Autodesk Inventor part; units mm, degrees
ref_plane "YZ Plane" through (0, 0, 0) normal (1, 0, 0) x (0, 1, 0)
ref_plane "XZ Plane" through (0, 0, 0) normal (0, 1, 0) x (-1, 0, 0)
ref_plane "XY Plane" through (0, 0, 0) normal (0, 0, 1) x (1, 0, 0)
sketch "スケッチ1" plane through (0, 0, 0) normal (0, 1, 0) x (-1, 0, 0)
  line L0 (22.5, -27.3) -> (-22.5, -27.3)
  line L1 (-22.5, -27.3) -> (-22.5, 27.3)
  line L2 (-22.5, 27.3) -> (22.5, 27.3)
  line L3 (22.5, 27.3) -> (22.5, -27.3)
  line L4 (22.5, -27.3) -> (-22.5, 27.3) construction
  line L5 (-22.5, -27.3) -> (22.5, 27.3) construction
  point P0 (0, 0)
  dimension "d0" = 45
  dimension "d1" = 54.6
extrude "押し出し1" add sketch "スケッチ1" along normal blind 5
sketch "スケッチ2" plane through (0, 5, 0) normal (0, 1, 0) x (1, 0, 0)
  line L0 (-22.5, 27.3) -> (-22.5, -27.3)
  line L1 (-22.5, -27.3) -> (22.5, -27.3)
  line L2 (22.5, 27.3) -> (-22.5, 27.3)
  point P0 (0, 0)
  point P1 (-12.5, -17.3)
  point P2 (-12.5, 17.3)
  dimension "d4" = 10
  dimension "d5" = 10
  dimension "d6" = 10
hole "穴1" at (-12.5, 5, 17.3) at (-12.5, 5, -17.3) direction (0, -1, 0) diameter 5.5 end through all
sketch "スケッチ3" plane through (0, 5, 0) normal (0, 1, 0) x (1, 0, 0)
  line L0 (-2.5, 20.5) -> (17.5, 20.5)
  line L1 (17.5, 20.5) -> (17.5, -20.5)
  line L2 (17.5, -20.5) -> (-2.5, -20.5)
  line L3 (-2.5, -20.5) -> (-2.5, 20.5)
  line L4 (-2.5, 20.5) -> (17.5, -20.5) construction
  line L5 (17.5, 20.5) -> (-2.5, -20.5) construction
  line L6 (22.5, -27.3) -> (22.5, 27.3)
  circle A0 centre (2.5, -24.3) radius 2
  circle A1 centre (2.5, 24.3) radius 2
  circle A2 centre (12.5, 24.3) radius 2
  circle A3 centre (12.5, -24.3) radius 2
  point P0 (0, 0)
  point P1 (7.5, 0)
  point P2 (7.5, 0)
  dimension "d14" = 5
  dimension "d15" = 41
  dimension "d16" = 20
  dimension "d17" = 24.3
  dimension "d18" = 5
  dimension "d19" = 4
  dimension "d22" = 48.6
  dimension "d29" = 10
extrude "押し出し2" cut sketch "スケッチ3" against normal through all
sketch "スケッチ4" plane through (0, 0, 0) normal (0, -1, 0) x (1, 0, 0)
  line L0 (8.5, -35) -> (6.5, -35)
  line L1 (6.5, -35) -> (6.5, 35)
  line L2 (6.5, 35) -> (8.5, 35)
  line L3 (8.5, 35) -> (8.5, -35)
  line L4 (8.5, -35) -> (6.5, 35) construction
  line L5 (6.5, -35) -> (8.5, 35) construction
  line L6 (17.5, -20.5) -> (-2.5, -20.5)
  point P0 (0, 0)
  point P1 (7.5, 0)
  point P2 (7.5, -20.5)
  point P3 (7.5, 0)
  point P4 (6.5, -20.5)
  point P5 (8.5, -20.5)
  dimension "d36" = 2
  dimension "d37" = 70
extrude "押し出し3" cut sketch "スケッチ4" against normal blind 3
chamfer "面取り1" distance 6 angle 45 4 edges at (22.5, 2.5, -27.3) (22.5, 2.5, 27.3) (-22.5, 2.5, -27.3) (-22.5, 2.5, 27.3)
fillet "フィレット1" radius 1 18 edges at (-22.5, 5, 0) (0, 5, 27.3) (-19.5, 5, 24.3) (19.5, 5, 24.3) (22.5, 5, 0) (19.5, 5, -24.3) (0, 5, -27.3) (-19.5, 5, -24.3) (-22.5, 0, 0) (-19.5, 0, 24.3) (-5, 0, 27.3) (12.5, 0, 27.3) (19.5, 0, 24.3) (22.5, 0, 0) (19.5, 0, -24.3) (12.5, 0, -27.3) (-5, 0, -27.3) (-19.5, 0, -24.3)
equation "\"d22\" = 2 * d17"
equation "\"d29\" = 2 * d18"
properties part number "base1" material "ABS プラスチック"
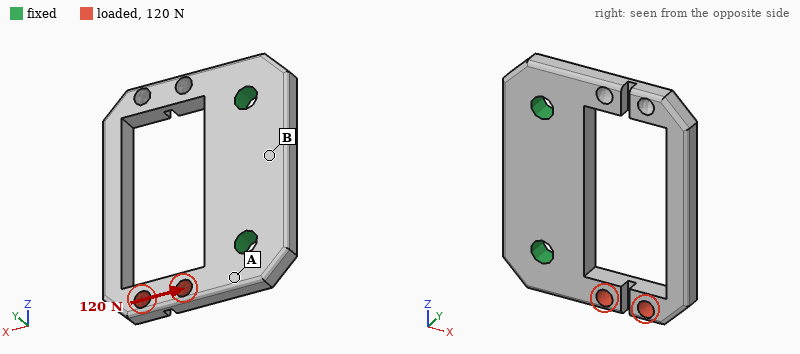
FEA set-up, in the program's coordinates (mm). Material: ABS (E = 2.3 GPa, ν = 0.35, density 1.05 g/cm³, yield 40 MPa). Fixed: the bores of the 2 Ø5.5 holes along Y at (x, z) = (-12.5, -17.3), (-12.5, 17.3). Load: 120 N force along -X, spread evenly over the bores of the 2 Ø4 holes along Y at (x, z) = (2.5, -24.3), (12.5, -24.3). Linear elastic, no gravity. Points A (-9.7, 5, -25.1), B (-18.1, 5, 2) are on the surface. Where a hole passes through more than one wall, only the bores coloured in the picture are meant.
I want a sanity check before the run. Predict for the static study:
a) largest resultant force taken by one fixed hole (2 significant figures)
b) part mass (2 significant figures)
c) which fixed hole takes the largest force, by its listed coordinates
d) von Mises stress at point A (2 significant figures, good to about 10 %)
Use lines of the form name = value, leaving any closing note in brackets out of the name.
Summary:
largest resultant force taken by one fixed hole = 130 N
part mass = 7.5 g
which fixed hole takes the largest force, by its listed coordinates = (-12.5, -17.3)
von Mises stress at point A = 2.7 MPa
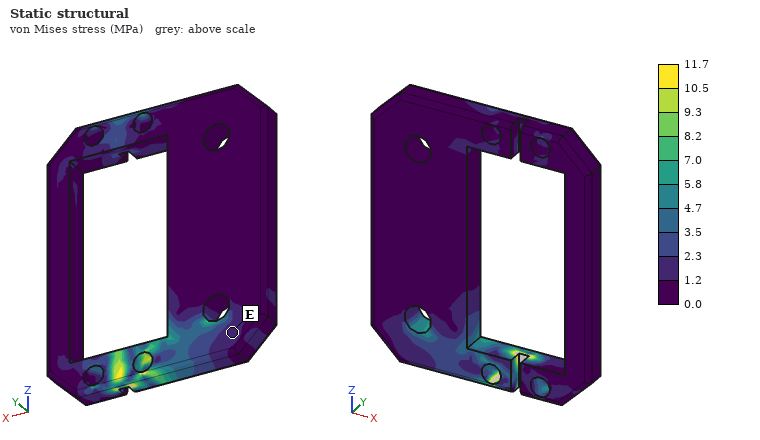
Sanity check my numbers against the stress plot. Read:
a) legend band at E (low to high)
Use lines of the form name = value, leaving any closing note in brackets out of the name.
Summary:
legend band at E = 1.2 to 2.3 MPa
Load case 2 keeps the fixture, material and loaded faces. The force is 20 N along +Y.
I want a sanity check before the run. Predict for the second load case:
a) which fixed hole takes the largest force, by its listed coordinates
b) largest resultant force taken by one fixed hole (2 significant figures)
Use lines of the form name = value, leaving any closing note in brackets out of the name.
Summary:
which fixed hole takes the largest force, by its listed coordinates = (-12.5, -17.3)
largest resultant force taken by one fixed hole = 21 N
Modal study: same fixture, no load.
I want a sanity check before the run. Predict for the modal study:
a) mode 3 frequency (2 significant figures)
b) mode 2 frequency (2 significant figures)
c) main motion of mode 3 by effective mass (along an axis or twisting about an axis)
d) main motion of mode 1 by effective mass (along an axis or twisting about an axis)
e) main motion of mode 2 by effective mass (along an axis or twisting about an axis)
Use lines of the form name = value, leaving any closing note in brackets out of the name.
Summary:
mode 3 frequency = 1400 Hz
mode 2 frequency = 1300 Hz
main motion of mode 3 by effective mass = along Z
main motion of mode 1 by effective mass = along Y
main motion of mode 2 by effective mass = twisting about X
